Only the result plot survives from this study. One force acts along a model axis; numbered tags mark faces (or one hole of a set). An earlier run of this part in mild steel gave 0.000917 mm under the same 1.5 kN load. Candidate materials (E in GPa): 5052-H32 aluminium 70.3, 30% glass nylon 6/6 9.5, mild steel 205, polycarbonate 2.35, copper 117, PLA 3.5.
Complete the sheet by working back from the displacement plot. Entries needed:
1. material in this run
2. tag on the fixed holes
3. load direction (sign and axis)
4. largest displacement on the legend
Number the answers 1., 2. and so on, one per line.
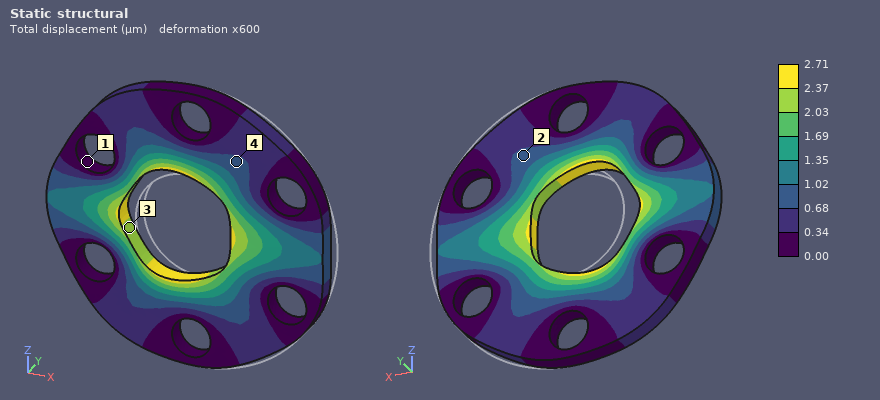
1. 5052-H32 aluminium
2. 1
3. -X
4. 2.71 µm
